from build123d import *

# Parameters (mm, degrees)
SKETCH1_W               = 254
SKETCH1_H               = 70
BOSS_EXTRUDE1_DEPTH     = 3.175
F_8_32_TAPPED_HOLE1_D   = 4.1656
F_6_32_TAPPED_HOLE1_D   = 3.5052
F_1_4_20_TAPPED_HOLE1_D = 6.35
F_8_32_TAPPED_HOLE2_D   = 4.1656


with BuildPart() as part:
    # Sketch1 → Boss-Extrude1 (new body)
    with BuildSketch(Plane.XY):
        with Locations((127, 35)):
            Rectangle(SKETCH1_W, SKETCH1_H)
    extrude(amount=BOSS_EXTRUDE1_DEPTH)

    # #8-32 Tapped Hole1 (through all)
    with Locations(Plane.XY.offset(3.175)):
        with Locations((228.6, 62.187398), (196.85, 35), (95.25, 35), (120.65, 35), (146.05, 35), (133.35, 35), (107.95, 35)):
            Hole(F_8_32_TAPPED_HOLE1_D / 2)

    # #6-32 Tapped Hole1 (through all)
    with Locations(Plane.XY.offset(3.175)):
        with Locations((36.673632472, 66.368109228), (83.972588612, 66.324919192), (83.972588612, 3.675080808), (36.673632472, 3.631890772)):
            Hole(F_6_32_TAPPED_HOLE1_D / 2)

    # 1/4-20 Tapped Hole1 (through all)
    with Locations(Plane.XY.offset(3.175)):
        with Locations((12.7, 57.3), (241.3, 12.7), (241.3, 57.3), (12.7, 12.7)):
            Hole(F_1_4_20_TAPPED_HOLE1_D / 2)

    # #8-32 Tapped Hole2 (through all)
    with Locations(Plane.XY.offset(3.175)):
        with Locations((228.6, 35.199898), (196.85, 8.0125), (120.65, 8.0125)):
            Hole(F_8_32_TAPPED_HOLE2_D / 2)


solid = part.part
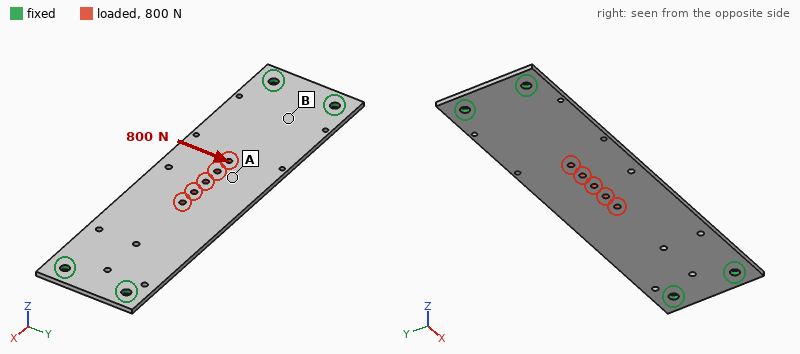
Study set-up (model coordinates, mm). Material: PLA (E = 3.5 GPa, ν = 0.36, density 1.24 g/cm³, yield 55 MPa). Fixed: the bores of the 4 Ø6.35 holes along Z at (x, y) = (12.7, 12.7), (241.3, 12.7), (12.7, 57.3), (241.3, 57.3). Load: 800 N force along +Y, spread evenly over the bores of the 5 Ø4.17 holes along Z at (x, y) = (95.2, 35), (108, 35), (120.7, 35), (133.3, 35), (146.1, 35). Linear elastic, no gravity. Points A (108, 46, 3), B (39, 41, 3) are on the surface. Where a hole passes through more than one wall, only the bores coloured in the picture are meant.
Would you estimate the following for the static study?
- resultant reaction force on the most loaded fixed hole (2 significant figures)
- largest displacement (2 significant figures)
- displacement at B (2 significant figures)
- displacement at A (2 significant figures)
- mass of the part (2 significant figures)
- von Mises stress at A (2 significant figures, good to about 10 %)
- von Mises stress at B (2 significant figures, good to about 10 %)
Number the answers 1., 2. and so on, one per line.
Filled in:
1. 510 N
2. 0.35 mm
3. 0.079 mm
4. 0.33 mm
5. 69 g
6. 3.1 MPa
7. 5.3 MPa
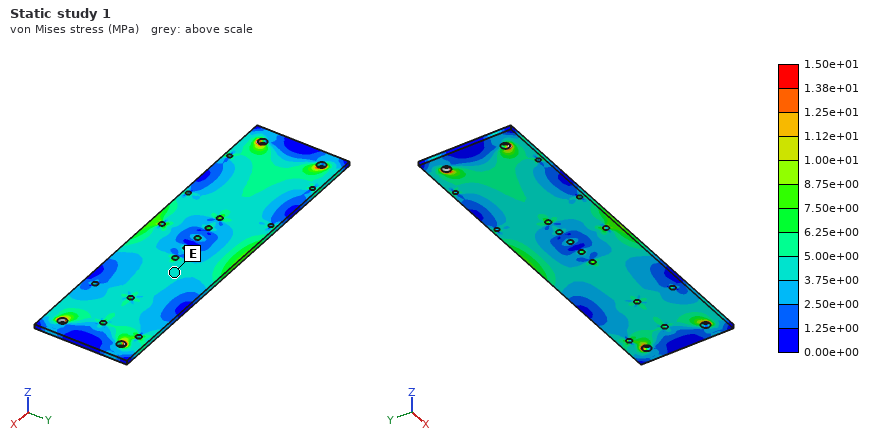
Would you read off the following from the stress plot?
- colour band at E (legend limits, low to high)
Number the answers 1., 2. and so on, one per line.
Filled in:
1. 3.75e+00 to 5.00e+00 MPa
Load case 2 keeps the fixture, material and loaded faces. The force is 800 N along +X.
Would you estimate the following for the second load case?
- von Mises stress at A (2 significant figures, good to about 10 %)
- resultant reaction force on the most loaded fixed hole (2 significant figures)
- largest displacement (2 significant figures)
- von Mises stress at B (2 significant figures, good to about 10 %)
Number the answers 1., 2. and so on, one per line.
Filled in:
1. 2.2 MPa
2. 210 N
3. 76 µm
4. 1.7 MPa
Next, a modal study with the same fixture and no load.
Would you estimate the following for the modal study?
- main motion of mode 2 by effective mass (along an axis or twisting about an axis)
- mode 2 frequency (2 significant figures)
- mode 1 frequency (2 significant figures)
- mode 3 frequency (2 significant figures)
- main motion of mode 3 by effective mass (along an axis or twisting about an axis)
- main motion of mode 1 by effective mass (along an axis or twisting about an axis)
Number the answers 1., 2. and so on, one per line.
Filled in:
1. twisting about X
2. 240 Hz
3. 110 Hz
4. 300 Hz
5. twisting about Y
6. along Z
